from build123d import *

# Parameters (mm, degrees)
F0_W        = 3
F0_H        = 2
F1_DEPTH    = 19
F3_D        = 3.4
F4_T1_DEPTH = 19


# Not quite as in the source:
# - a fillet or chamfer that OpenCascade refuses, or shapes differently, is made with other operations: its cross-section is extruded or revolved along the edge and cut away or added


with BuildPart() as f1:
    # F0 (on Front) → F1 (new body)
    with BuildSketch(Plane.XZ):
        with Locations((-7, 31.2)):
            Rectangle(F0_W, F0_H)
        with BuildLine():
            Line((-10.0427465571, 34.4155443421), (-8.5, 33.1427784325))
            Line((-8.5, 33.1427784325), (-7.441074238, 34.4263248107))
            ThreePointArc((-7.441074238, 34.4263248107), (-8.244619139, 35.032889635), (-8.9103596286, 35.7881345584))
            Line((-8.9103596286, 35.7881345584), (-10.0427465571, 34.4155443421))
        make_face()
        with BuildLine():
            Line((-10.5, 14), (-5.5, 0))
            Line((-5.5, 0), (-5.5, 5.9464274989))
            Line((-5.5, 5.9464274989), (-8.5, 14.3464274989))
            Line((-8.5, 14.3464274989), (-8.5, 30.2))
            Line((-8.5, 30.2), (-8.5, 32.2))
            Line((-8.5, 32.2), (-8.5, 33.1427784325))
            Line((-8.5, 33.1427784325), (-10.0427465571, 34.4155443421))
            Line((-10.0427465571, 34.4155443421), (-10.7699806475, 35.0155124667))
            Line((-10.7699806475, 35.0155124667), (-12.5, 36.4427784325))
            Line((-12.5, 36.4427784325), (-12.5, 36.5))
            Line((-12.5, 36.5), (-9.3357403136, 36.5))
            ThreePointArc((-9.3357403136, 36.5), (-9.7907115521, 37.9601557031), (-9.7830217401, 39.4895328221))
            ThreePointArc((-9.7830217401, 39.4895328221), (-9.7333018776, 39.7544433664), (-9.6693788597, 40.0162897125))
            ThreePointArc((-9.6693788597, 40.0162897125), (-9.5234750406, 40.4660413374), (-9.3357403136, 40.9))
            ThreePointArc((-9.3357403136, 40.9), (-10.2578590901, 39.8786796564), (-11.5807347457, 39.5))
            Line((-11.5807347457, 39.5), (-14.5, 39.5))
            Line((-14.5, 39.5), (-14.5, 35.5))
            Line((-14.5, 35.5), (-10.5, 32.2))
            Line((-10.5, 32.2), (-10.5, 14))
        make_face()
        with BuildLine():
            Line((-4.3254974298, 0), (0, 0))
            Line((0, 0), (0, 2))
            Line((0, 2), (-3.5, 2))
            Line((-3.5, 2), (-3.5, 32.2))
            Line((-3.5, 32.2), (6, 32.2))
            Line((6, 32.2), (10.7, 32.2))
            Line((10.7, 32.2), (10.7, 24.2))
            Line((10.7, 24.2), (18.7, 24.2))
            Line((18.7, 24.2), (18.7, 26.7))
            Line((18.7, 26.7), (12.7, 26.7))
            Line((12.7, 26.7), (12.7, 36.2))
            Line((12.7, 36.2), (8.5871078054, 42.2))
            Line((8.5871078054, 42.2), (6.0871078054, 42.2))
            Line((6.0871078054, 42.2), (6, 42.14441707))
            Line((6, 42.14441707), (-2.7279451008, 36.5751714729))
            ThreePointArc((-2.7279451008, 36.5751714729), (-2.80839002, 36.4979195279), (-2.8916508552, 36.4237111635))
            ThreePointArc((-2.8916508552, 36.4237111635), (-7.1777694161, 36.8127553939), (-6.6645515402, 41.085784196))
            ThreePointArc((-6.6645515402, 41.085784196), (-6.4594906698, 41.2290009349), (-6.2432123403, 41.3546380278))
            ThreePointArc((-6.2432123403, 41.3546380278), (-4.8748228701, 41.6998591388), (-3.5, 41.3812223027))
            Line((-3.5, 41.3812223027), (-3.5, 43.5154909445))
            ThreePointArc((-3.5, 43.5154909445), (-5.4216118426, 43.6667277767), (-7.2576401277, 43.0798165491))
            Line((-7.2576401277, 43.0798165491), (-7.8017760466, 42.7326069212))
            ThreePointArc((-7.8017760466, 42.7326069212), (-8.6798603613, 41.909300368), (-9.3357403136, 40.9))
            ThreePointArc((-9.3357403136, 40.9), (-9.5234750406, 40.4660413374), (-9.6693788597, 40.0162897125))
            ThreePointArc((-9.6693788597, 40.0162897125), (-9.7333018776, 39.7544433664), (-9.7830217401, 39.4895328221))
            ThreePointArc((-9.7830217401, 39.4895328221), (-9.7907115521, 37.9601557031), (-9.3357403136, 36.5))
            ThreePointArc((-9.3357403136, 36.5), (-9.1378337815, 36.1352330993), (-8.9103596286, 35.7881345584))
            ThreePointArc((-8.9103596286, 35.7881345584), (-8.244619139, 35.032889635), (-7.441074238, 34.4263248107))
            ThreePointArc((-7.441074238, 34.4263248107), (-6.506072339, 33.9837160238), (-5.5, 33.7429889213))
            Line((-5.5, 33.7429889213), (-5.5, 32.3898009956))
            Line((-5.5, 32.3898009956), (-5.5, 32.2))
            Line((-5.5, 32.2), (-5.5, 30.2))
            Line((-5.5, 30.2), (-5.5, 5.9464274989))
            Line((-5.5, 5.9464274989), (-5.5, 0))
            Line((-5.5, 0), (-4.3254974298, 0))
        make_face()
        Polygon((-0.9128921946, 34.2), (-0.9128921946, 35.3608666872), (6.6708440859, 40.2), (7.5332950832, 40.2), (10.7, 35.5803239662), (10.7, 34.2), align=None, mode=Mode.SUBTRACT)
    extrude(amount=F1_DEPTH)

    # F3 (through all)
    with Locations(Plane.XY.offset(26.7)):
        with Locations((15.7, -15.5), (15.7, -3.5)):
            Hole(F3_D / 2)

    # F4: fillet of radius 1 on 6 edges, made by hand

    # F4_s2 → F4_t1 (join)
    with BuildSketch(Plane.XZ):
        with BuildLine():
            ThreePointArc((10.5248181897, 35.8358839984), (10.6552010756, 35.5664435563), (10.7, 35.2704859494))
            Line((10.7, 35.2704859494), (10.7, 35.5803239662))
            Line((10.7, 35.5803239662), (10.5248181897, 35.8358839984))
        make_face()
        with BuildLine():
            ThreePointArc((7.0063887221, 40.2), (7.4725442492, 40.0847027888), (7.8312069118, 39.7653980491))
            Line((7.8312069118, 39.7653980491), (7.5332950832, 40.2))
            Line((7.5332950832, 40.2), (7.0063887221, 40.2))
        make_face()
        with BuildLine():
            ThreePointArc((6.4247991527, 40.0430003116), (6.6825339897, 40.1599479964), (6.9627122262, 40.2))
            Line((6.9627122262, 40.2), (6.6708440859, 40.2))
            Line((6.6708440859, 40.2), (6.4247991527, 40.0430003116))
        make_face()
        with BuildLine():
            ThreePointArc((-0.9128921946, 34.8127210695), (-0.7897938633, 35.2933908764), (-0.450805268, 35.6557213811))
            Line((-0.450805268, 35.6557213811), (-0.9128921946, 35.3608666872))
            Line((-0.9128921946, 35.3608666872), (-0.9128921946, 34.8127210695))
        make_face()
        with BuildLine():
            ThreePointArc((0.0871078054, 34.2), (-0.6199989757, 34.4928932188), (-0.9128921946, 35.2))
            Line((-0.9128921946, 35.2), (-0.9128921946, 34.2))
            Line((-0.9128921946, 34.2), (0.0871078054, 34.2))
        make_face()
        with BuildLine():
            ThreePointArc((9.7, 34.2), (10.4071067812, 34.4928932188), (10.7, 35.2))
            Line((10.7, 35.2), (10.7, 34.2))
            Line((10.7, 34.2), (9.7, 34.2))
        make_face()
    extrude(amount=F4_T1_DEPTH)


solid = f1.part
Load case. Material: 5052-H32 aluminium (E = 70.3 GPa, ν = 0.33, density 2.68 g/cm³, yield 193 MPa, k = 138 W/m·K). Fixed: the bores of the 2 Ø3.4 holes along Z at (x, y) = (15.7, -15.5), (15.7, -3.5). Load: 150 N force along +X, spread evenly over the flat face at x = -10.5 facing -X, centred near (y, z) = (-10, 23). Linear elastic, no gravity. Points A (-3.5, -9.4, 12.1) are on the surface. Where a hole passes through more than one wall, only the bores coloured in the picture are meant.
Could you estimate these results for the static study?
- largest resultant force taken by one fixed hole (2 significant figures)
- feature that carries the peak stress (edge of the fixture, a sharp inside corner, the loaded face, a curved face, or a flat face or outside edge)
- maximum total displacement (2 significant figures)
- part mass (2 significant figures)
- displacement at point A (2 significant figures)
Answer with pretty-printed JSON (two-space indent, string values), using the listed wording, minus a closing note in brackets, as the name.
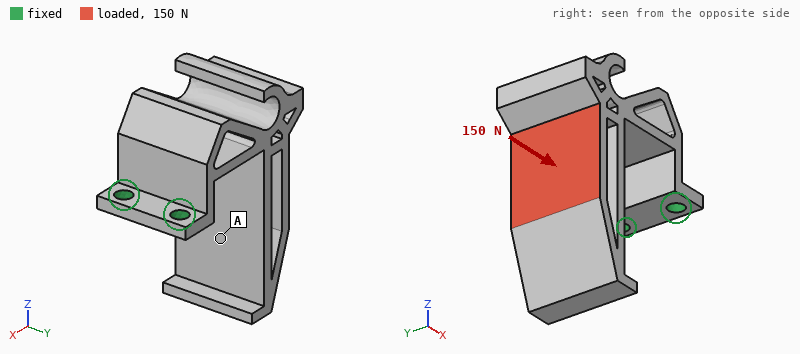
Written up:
{
  "largest resultant force taken by one fixed hole": "75 N",
  "feature that carries the peak stress": "a flat face or outside edge",
  "maximum total displacement": "0.45 mm",
  "part mass": "16 g",
  "displacement at point A": "0.30 mm"
}
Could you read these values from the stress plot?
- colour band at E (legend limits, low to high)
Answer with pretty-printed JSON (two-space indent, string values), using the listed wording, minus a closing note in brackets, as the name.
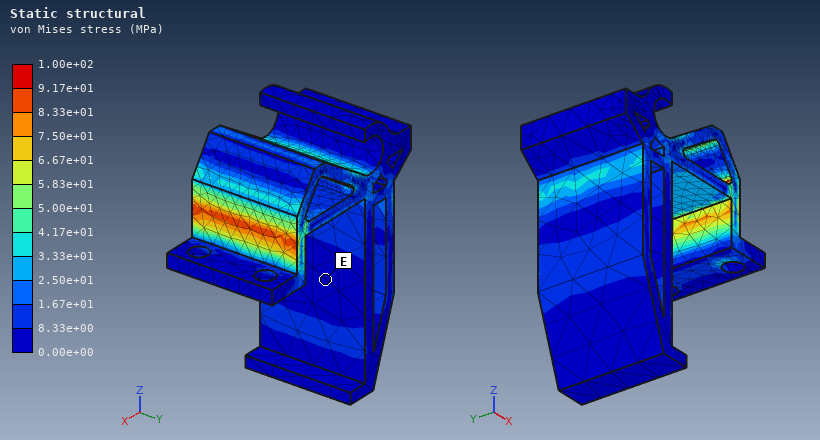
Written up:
{
  "colour band at E": "0.00e+00 to 8.33e+00 MPa"
}
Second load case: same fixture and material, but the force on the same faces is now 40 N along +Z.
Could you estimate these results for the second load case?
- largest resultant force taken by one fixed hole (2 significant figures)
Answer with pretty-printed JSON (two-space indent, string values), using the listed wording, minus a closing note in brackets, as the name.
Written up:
{
  "largest resultant force taken by one fixed hole": "20 N"
}
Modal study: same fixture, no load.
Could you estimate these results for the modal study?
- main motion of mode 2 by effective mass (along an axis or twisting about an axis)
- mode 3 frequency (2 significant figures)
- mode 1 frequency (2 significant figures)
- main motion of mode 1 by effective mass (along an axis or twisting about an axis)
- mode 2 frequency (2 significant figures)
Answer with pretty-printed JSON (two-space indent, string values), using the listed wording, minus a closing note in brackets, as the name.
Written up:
{
  "main motion of mode 2 by effective mass": "along Y",
  "mode 3 frequency": "2400 Hz",
  "mode 1 frequency": "610 Hz",
  "main motion of mode 1 by effective mass": "along Z",
  "mode 2 frequency": "1600 Hz"
}
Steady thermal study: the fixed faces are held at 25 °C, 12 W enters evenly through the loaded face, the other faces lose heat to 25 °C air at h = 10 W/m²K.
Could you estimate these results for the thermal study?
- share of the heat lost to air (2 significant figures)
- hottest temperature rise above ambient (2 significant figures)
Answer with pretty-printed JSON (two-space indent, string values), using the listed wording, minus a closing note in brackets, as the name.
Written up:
{
  "share of the heat lost to air": "16 %",
  "hottest temperature rise above ambient": "52 K"
}
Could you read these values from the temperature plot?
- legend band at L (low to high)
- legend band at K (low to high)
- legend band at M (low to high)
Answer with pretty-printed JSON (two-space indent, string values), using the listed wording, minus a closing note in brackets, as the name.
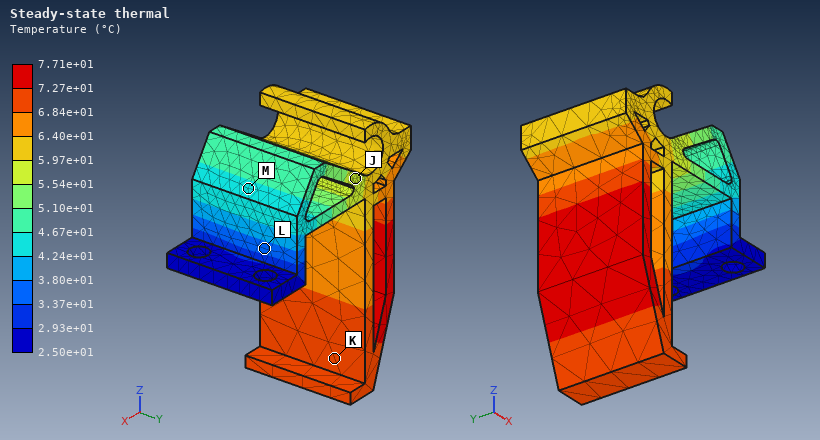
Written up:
{
  "legend band at L": "3.37e+01 to 3.80e+01 °C",
  "legend band at K": "6.84e+01 to 7.27e+01 °C",
  "legend band at M": "4.24e+01 to 4.67e+01 °C"
}
